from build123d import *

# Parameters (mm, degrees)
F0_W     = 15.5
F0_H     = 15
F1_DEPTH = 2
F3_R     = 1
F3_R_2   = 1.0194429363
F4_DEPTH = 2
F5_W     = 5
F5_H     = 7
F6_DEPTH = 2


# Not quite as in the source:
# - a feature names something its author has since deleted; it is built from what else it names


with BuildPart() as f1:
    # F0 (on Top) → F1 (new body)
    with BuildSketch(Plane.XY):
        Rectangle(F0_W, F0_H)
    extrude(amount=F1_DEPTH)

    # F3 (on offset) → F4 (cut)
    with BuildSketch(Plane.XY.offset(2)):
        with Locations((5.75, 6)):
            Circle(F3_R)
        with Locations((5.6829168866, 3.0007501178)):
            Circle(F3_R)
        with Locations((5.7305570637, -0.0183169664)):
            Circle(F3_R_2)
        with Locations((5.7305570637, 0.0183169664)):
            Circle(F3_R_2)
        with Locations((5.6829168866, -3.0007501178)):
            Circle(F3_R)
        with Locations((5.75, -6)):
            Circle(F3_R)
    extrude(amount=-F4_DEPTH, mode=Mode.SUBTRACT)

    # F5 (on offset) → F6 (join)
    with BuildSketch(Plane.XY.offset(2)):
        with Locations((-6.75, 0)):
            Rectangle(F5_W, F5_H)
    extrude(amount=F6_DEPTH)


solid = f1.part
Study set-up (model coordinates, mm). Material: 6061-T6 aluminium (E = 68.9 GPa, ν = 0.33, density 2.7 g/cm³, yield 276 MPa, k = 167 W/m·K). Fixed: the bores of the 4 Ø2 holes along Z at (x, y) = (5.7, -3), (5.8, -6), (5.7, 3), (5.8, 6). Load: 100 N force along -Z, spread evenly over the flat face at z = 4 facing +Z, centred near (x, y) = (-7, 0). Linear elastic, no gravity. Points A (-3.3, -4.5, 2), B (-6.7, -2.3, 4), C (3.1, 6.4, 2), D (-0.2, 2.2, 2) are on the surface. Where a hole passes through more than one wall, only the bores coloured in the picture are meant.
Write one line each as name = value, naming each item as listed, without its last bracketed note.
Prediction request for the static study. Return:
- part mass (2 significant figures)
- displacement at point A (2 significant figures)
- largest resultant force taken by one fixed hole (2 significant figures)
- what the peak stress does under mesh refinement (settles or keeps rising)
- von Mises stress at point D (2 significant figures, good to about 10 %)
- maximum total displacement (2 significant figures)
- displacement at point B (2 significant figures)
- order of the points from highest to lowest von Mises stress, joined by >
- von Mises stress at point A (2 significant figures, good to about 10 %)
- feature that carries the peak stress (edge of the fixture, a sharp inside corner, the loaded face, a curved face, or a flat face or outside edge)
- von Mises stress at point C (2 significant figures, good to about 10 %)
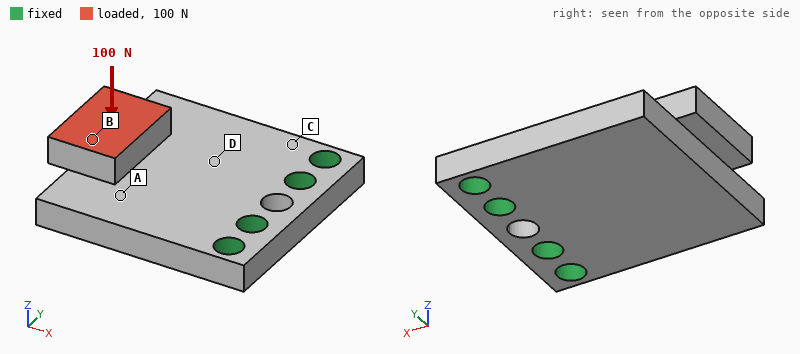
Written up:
part mass = 1.4 g
displacement at point A = 0.047 mm
largest resultant force taken by one fixed hole = 45 N
what the peak stress does under mesh refinement = keeps rising
von Mises stress at point D = 60 MPa
maximum total displacement = 0.11 mm
displacement at point B = 0.086 mm
order of the points from highest to lowest von Mises stress, joined by > = C > D > A > B
von Mises stress at point A = 33 MPa
feature that carries the peak stress = edge of the fixture
von Mises stress at point C = 98 MPa
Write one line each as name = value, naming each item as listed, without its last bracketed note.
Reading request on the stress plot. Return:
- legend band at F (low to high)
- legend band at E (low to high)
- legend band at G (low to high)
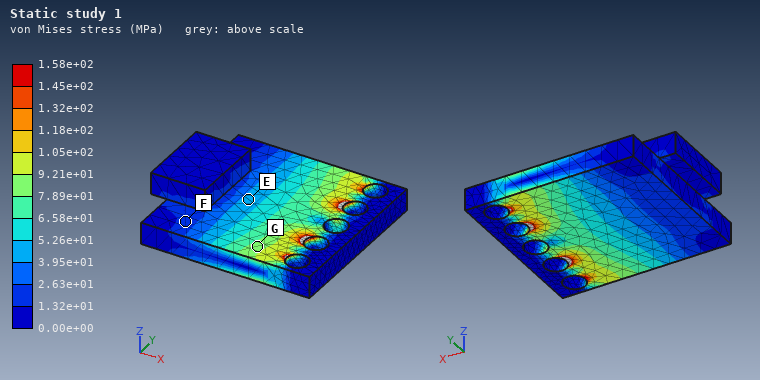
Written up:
legend band at F = 1.32e+01 to 2.63e+01 MPa
legend band at E = 3.95e+01 to 5.26e+01 MPa
legend band at G = 7.89e+01 to 9.21e+01 MPa
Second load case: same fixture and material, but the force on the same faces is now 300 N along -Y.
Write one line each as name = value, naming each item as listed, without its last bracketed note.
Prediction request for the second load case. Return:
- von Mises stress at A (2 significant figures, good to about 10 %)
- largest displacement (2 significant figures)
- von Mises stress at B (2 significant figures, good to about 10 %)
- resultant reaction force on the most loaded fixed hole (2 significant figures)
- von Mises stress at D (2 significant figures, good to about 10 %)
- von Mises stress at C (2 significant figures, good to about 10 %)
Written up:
von Mises stress at A = 73 MPa
largest displacement = 45 µm
von Mises stress at B = 33 MPa
resultant reaction force on the most loaded fixed hole = 260 N
von Mises stress at D = 77 MPa
von Mises stress at C = 41 MPa
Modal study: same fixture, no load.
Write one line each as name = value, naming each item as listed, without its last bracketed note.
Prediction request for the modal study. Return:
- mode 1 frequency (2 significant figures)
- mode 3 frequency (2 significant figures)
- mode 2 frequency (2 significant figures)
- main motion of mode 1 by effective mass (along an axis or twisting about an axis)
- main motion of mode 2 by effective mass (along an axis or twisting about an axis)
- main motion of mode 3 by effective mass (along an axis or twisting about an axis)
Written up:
mode 1 frequency = 7700 Hz
mode 3 frequency = 37 kHz
mode 2 frequency = 20 kHz
main motion of mode 1 by effective mass = along Z
main motion of mode 2 by effective mass = twisting about X
main motion of mode 3 by effective mass = along Y
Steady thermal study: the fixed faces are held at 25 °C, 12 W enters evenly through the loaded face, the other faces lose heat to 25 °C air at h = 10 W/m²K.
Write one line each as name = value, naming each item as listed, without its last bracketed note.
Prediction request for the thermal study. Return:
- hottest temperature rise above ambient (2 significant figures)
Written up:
hottest temperature rise above ambient = 36 K
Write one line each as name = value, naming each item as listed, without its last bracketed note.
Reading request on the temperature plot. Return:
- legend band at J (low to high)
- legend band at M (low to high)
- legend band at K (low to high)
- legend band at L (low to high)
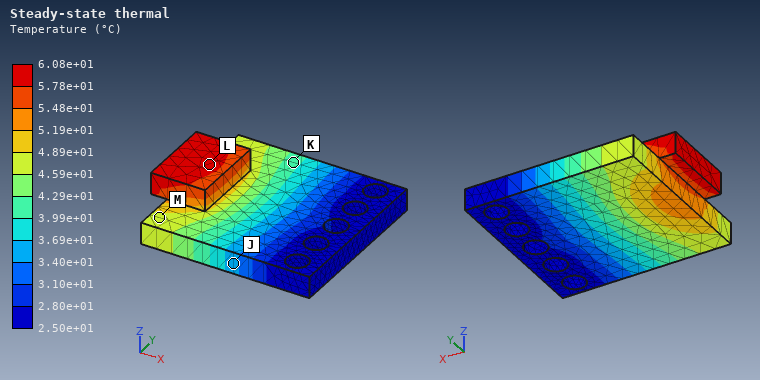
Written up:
legend band at J = 3.40e+01 to 3.69e+01 °C
legend band at M = 4.59e+01 to 4.89e+01 °C
legend band at K = 3.99e+01 to 4.29e+01 °C
legend band at L = 5.78e+01 to 6.08e+01 °C
